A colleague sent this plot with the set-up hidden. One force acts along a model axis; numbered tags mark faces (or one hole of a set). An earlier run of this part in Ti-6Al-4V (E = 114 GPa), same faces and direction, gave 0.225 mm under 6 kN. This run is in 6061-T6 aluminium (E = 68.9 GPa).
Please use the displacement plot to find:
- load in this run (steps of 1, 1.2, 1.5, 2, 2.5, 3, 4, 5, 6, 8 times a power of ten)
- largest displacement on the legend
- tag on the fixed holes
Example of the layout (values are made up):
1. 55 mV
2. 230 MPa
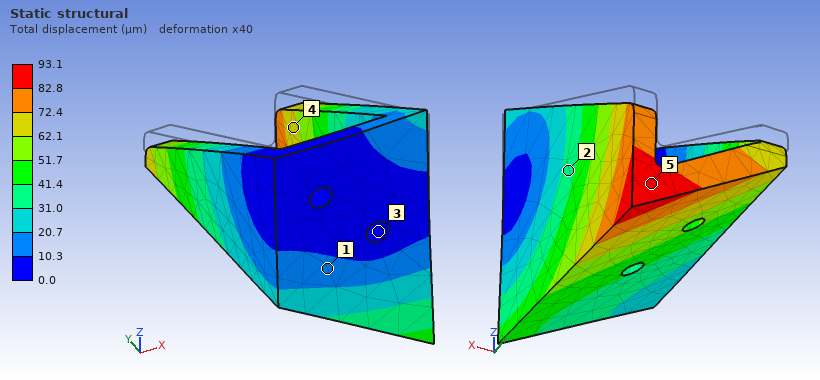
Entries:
1. 1.5 kN
2. 93.1 µm
3. 3
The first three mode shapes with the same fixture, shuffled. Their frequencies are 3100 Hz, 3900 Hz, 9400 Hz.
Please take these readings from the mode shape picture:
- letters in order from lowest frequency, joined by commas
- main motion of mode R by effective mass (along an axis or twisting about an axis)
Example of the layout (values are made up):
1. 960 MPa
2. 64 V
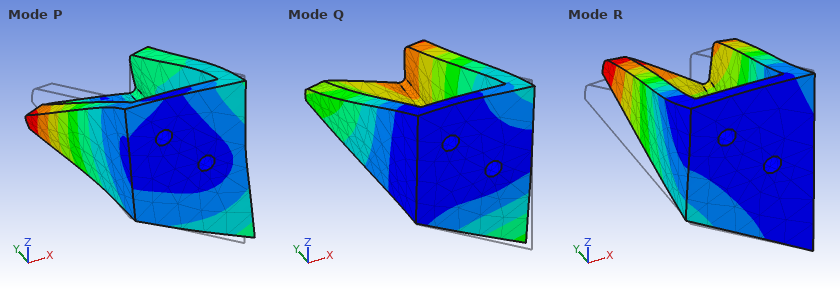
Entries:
1. R, Q, P
2. along X
